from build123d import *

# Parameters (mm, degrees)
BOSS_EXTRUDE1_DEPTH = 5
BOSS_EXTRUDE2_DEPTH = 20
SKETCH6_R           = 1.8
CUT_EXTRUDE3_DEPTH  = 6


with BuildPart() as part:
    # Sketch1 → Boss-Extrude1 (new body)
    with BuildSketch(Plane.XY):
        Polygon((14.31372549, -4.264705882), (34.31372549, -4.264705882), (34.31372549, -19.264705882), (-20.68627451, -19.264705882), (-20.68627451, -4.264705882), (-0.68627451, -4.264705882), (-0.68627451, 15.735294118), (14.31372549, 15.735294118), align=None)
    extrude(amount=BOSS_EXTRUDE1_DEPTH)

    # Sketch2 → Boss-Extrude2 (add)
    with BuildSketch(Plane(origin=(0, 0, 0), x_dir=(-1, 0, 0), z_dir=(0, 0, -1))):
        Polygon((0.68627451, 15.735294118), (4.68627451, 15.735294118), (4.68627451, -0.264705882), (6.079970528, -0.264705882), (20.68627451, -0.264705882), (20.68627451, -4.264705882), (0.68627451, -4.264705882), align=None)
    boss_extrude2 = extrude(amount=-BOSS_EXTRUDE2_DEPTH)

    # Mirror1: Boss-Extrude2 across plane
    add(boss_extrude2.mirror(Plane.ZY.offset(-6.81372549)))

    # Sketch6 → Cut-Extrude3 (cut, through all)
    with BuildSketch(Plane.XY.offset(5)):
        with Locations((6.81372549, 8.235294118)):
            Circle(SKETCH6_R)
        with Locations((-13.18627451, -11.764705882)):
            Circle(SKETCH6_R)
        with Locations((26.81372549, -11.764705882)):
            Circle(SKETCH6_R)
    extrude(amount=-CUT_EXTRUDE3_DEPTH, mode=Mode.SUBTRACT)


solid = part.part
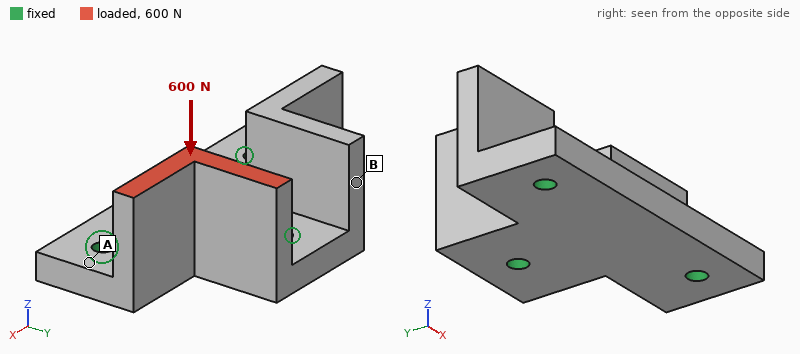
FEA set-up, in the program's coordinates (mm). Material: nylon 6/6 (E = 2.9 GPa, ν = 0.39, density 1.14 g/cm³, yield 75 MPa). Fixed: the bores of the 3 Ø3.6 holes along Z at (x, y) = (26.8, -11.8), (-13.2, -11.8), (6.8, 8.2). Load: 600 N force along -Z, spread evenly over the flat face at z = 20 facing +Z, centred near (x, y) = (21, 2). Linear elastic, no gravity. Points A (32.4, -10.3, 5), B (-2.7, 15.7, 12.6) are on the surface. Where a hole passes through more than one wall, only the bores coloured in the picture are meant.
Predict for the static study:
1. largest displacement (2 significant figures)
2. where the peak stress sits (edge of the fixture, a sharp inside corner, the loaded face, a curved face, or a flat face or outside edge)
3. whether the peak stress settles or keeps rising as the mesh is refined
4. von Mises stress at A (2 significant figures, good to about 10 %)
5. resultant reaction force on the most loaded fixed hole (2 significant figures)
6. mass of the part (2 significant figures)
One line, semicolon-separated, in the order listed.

0.33 mm; edge of the fixture; keeps rising; 13 MPa; 320 N; 13 g
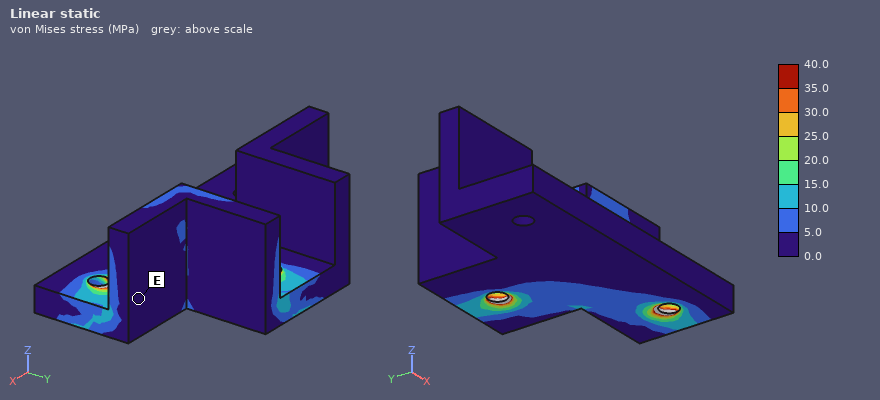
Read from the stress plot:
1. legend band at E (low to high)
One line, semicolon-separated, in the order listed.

0.0 to 5.0 MPa
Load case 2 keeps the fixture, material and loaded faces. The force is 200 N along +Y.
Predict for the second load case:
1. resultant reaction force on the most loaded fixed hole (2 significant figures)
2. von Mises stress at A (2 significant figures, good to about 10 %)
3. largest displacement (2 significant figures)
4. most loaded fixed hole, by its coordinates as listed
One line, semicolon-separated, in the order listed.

160 N; 5.8 MPa; 0.50 mm; (6.8, 8.2)
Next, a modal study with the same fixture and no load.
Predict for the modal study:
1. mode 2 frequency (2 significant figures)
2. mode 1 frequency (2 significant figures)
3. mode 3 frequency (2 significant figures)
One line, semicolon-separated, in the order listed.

3300 Hz; 3100 Hz; 4400 Hz
